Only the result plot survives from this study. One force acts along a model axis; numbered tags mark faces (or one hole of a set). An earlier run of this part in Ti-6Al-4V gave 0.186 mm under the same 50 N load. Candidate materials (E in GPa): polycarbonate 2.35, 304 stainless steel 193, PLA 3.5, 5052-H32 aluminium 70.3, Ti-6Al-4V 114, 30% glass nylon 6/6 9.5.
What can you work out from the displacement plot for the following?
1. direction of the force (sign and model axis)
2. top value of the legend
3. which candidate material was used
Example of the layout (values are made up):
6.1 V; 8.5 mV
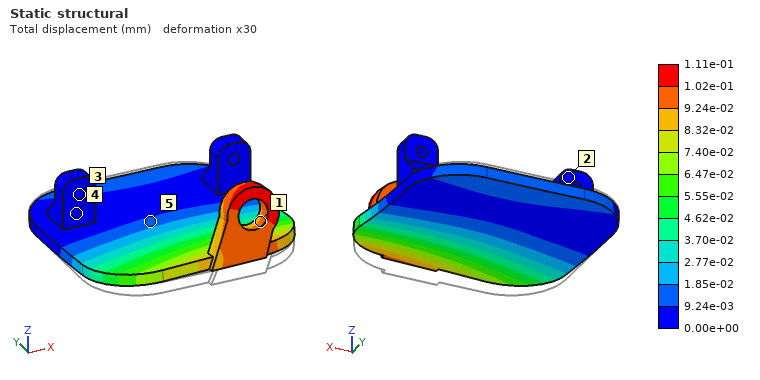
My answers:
+Z; 1.11e-01 mm; 304 stainless steel
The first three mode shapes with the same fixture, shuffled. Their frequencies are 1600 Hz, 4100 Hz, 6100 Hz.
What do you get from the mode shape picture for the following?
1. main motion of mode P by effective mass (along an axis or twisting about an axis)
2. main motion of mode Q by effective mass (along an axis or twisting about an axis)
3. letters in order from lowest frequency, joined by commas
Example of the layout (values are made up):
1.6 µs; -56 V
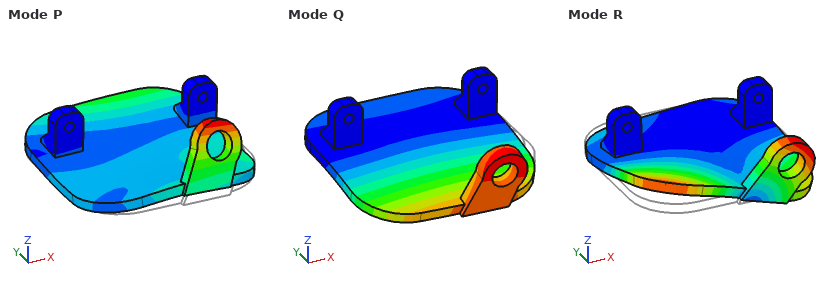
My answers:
along Y; along Z; Q, R, P
